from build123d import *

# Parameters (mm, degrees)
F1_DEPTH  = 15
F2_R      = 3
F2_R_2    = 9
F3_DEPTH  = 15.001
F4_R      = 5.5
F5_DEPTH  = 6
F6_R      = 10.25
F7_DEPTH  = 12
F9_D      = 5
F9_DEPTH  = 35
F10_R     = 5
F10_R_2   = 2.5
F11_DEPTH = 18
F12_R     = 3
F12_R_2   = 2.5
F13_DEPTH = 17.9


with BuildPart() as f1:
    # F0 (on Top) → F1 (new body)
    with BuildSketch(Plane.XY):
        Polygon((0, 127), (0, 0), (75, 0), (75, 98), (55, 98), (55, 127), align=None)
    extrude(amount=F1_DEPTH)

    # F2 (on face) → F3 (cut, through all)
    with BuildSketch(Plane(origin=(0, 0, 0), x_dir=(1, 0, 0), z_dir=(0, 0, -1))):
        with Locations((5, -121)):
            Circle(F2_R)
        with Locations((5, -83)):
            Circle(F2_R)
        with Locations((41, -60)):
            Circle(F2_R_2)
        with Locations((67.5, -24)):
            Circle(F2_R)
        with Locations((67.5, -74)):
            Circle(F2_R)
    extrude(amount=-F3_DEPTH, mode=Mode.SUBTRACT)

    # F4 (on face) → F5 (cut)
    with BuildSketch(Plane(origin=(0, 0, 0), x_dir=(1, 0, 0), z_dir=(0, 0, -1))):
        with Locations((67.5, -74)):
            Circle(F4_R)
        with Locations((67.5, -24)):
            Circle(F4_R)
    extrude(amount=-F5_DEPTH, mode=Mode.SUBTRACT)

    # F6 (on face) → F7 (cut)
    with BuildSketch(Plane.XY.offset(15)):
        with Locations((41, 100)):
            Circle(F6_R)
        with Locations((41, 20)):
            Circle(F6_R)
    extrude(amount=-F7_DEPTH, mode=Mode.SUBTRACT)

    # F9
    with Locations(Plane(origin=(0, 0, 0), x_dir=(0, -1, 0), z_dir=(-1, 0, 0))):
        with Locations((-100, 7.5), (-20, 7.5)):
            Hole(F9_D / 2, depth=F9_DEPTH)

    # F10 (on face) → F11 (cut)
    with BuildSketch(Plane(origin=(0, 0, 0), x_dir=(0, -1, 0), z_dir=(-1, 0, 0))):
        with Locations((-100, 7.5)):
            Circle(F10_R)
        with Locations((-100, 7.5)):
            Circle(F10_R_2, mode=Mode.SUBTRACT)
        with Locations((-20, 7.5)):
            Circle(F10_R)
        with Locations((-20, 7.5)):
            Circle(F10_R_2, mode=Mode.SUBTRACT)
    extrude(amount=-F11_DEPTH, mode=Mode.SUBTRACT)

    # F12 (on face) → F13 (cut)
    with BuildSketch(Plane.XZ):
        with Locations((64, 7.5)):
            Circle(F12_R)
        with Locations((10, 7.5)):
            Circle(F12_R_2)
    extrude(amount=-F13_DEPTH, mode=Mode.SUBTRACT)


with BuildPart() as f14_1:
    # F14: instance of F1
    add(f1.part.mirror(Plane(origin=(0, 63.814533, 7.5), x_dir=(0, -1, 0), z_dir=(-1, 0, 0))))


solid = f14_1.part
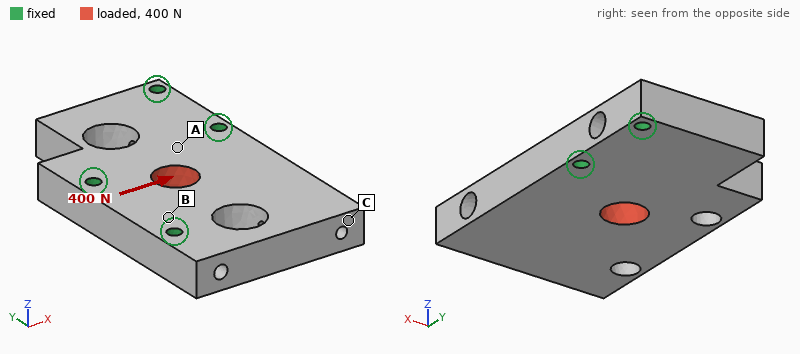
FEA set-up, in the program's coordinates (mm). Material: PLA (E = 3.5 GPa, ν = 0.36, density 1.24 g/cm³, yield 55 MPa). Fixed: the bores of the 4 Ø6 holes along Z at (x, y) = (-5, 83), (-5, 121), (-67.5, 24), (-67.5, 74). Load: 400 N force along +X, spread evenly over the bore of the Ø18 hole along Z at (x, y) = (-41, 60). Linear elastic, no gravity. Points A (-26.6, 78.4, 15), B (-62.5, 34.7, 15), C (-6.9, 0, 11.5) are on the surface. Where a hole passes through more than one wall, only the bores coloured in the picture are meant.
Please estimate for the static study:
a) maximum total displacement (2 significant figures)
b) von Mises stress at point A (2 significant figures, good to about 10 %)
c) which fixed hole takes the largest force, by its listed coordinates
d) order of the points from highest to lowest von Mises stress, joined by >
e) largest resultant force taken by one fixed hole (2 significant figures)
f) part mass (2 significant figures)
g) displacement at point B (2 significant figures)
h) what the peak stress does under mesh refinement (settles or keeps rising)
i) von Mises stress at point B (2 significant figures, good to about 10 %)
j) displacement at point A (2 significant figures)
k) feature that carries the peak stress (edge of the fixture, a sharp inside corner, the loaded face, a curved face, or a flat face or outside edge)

8.0 µm
0.30 MPa
(-67.5, 74)
B > A > C
170 N
140 g
2.5 µm
keeps rising
0.47 MPa
3.0 µm
edge of the fixture
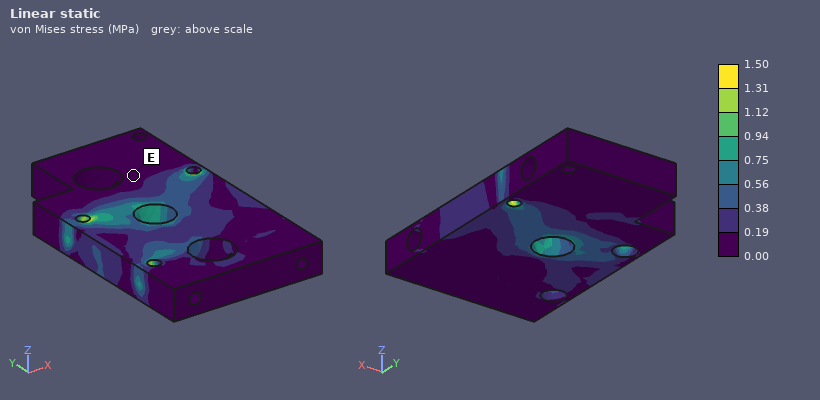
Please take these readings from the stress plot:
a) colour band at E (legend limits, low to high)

0.00 to 0.19 MPa
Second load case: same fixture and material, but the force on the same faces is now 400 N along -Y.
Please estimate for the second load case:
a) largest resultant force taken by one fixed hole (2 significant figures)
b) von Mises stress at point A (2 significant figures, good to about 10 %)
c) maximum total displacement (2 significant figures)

140 N
0.34 MPa
7.0 µm
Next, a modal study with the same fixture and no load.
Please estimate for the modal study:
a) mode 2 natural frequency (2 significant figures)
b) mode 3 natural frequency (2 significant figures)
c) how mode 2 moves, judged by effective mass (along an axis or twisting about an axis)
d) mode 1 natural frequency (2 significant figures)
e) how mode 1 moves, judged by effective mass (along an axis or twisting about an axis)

2400 Hz
3000 Hz
along Z
1100 Hz
along Z
